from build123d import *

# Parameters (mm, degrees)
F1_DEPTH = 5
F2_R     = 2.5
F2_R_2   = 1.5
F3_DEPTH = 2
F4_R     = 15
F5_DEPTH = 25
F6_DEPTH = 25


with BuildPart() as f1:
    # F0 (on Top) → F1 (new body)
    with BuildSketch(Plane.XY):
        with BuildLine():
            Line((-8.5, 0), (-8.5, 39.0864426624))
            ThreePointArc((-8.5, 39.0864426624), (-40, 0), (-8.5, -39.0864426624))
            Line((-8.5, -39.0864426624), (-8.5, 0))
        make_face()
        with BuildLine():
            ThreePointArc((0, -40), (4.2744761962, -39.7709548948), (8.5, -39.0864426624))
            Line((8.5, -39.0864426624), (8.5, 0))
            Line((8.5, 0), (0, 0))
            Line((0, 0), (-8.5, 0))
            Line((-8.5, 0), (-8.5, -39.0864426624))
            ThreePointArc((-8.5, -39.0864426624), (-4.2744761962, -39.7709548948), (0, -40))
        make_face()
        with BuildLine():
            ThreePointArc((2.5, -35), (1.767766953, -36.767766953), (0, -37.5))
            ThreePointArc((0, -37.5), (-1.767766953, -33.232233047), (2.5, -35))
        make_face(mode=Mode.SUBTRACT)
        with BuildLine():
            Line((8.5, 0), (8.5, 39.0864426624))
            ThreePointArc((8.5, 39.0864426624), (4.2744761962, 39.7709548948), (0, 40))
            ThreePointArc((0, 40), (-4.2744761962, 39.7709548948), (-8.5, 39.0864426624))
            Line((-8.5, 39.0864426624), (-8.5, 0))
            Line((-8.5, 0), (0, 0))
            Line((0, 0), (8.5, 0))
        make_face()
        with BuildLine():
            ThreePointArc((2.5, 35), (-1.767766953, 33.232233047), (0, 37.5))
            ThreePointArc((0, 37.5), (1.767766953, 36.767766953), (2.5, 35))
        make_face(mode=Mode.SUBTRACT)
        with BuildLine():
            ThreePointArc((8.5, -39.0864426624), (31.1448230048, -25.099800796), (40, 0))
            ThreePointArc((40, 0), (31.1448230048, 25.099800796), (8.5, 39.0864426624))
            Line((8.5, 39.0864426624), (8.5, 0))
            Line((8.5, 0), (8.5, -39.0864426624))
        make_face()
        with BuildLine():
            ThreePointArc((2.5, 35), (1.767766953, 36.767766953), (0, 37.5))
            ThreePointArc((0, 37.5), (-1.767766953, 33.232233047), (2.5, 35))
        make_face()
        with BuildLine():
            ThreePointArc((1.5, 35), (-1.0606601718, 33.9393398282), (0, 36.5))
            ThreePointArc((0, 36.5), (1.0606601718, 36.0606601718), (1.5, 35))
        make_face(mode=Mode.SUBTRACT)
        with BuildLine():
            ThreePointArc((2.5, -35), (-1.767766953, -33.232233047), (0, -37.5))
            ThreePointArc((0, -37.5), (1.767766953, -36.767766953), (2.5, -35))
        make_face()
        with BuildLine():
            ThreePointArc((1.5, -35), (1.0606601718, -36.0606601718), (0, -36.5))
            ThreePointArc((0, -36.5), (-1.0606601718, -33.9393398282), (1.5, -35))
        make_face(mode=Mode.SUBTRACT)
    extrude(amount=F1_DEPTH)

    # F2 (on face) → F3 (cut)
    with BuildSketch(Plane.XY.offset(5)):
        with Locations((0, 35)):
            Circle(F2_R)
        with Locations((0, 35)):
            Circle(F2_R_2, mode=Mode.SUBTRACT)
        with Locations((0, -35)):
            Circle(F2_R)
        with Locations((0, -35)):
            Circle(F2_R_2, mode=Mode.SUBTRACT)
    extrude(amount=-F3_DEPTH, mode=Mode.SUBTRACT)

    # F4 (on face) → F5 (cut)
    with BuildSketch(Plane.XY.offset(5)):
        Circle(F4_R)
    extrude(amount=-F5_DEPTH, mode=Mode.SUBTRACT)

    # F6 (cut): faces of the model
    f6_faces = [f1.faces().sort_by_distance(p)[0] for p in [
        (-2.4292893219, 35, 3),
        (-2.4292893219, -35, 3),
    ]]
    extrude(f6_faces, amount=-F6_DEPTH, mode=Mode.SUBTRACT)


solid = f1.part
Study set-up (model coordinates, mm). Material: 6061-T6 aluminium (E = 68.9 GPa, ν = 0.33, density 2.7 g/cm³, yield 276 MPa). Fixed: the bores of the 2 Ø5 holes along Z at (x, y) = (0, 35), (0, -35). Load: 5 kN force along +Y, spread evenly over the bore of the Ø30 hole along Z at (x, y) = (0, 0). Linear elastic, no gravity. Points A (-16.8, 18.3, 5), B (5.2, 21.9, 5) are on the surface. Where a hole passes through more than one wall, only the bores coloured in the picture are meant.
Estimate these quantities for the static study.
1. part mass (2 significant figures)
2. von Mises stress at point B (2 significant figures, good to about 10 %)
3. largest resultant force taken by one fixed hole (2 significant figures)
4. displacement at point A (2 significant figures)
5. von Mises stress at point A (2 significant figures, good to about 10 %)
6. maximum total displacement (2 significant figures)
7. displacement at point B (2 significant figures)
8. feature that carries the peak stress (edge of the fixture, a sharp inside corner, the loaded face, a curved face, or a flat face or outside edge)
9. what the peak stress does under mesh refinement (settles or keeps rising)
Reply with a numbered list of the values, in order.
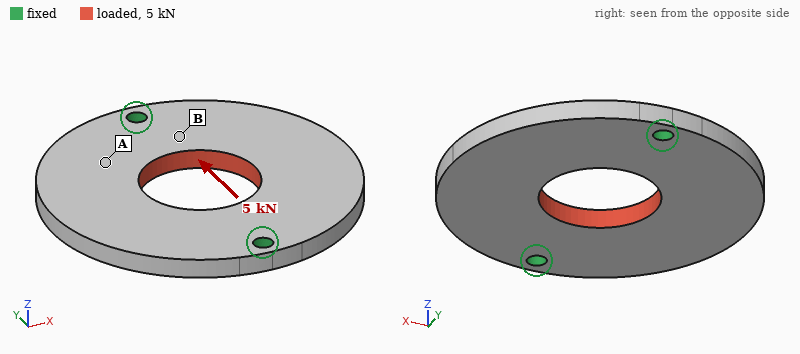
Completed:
1. 58 g
2. 22 MPa
3. 2.5 kN
4. 8.9 µm
5. 9.0 MPa
6. 12 µm
7. 5.7 µm
8. edge of the fixture
9. keeps rising
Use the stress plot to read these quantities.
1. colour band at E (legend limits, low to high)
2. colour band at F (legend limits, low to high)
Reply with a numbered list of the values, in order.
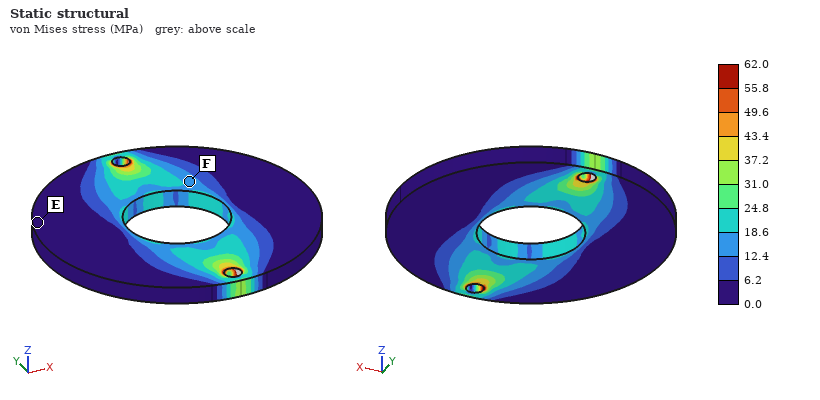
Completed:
1. 0.0 to 6.2 MPa
2. 12.4 to 18.6 MPa
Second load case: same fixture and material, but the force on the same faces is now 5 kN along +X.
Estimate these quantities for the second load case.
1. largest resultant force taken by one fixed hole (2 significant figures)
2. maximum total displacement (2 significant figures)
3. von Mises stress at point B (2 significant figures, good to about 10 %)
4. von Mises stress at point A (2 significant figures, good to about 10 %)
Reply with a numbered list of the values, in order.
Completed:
1. 2.5 kN
2. 14 µm
3. 16 MPa
4. 13 MPa
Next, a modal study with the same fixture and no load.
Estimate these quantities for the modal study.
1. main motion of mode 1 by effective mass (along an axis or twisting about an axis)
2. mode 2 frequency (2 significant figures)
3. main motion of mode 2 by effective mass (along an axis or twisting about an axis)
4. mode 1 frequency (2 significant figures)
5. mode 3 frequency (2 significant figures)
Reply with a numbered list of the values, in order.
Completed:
1. twisting about Y
2. 2500 Hz
3. along Z
4. 1900 Hz
5. 5800 Hz
